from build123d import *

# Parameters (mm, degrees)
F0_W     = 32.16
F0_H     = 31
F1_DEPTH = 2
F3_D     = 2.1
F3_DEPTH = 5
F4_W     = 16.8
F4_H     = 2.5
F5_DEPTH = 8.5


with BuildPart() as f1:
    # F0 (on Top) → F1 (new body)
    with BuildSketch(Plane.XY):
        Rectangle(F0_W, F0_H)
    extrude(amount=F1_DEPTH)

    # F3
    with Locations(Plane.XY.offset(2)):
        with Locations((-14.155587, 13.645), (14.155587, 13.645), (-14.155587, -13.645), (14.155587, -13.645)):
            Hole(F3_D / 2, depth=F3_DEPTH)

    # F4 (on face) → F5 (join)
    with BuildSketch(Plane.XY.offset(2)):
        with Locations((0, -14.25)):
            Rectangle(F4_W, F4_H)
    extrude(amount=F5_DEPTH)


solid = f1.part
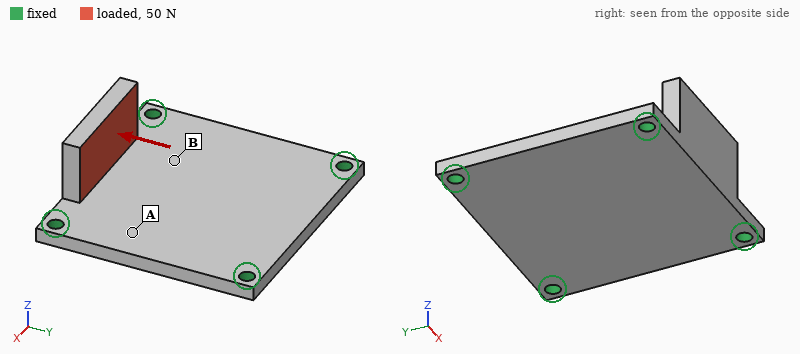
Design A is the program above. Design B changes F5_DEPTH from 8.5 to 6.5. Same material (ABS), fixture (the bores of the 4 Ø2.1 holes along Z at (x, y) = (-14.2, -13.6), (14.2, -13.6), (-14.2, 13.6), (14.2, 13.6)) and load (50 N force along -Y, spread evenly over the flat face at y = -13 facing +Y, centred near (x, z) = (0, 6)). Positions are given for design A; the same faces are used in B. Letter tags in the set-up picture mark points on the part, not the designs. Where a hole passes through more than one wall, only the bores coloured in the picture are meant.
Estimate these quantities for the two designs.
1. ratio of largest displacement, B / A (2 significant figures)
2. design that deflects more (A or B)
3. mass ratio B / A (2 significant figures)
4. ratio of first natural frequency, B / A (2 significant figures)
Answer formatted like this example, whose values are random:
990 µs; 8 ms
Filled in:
0.63; A; 0.96; 1.1
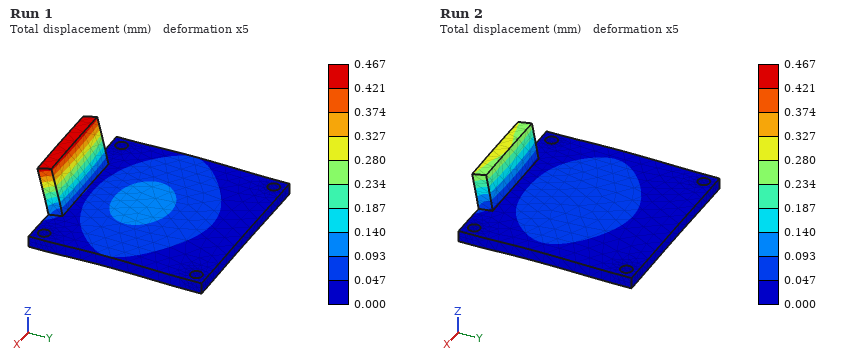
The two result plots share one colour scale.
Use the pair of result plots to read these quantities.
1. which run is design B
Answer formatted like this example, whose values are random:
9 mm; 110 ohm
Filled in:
Run 2
